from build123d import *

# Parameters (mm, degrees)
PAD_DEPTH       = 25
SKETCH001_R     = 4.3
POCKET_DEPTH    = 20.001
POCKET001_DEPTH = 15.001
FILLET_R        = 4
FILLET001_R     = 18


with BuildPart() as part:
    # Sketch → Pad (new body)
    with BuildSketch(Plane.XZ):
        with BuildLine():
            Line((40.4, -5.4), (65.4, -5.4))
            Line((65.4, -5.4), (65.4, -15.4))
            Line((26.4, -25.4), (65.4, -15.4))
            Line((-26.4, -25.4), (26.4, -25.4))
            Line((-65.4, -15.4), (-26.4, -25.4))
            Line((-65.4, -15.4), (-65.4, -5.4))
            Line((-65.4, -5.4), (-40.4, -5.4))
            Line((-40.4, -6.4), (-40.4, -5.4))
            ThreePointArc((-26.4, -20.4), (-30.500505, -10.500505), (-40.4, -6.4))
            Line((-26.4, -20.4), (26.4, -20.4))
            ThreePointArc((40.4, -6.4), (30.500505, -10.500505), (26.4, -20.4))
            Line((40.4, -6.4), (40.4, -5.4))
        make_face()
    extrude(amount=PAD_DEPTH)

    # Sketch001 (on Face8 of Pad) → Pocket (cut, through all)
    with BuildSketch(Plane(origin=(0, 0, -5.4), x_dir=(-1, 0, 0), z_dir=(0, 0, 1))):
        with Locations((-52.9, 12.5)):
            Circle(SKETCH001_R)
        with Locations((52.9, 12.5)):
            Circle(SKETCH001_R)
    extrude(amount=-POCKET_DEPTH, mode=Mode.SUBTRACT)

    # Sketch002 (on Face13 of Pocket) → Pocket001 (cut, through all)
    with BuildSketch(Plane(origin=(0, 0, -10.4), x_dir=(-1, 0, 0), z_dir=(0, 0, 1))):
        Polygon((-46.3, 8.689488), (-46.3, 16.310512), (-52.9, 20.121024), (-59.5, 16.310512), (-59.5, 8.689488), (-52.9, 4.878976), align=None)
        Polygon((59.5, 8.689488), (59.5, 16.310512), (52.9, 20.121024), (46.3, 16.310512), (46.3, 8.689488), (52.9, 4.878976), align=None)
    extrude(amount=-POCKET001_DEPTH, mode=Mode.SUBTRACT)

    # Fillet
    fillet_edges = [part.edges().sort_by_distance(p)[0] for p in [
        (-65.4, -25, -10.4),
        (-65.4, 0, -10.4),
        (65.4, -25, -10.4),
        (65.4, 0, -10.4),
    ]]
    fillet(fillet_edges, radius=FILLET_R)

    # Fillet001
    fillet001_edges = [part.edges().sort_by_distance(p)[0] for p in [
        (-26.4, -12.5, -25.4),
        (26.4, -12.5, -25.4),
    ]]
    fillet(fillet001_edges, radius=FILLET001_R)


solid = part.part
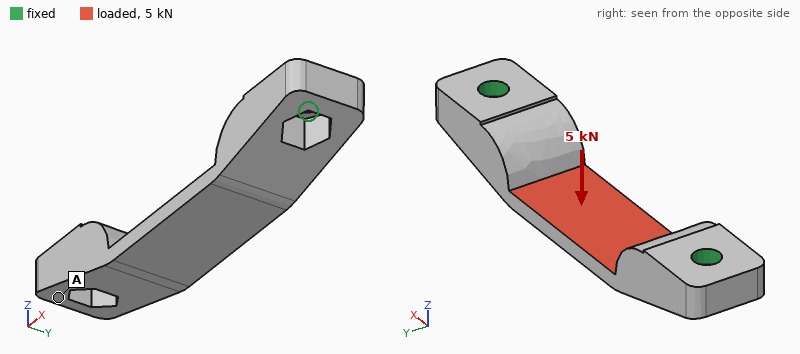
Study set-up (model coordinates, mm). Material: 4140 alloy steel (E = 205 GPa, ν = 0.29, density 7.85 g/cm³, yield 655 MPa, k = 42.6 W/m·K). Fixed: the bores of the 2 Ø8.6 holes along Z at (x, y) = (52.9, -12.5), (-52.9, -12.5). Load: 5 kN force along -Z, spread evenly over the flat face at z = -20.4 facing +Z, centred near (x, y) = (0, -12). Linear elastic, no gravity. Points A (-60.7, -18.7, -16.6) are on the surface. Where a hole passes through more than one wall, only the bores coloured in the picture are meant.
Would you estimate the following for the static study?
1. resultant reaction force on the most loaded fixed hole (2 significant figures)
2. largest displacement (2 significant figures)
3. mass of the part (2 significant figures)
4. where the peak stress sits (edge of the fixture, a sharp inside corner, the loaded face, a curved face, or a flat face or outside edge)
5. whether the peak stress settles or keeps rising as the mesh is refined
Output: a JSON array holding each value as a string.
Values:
["5.2 kN", "75 µm", "230 g", "edge of the fixture", "keeps rising"]
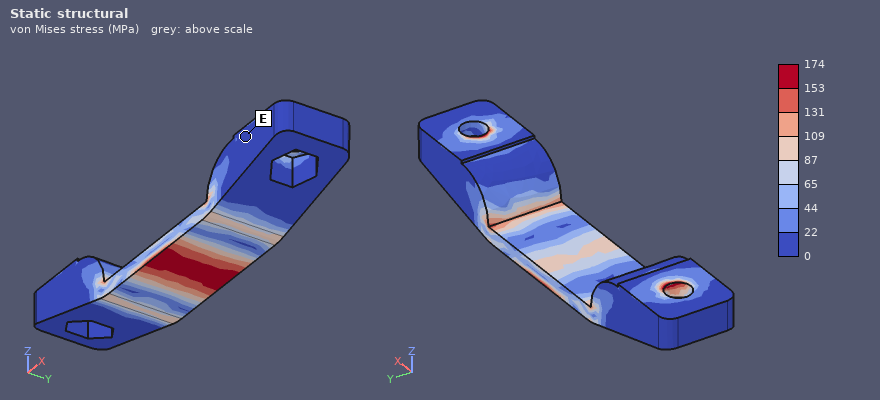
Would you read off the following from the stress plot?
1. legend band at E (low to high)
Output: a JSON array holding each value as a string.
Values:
["0 to 22 MPa"]
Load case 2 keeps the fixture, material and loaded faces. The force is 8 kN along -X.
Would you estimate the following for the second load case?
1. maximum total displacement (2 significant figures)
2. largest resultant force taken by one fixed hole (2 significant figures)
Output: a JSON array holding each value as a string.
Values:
["42 µm", "4.0 kN"]
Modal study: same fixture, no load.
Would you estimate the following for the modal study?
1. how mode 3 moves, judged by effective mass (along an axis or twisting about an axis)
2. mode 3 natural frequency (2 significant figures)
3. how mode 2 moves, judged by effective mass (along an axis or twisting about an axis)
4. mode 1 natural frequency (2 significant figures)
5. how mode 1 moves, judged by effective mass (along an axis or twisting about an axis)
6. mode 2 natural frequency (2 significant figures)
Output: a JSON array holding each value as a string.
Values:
["along Z", "6400 Hz", "along X", "5800 Hz", "along Y", "6100 Hz"]
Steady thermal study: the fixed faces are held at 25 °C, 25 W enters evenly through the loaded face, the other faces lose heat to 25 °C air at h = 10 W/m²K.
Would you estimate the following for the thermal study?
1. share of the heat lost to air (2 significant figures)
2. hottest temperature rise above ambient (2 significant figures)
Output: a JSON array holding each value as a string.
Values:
["7.7 %", "64 K"]
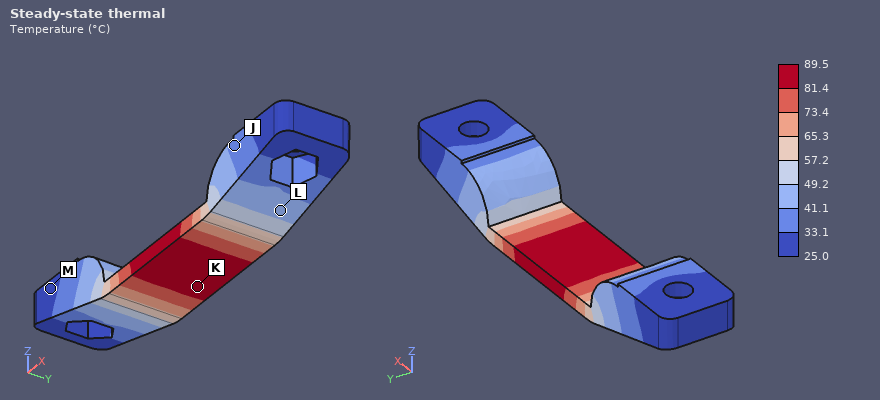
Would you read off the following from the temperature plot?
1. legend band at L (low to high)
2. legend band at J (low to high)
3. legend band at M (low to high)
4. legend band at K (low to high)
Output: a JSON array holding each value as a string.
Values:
["41.1 to 49.2 °C", "33.1 to 41.1 °C", "25.0 to 33.1 °C", "81.4 to 89.5 °C"]
